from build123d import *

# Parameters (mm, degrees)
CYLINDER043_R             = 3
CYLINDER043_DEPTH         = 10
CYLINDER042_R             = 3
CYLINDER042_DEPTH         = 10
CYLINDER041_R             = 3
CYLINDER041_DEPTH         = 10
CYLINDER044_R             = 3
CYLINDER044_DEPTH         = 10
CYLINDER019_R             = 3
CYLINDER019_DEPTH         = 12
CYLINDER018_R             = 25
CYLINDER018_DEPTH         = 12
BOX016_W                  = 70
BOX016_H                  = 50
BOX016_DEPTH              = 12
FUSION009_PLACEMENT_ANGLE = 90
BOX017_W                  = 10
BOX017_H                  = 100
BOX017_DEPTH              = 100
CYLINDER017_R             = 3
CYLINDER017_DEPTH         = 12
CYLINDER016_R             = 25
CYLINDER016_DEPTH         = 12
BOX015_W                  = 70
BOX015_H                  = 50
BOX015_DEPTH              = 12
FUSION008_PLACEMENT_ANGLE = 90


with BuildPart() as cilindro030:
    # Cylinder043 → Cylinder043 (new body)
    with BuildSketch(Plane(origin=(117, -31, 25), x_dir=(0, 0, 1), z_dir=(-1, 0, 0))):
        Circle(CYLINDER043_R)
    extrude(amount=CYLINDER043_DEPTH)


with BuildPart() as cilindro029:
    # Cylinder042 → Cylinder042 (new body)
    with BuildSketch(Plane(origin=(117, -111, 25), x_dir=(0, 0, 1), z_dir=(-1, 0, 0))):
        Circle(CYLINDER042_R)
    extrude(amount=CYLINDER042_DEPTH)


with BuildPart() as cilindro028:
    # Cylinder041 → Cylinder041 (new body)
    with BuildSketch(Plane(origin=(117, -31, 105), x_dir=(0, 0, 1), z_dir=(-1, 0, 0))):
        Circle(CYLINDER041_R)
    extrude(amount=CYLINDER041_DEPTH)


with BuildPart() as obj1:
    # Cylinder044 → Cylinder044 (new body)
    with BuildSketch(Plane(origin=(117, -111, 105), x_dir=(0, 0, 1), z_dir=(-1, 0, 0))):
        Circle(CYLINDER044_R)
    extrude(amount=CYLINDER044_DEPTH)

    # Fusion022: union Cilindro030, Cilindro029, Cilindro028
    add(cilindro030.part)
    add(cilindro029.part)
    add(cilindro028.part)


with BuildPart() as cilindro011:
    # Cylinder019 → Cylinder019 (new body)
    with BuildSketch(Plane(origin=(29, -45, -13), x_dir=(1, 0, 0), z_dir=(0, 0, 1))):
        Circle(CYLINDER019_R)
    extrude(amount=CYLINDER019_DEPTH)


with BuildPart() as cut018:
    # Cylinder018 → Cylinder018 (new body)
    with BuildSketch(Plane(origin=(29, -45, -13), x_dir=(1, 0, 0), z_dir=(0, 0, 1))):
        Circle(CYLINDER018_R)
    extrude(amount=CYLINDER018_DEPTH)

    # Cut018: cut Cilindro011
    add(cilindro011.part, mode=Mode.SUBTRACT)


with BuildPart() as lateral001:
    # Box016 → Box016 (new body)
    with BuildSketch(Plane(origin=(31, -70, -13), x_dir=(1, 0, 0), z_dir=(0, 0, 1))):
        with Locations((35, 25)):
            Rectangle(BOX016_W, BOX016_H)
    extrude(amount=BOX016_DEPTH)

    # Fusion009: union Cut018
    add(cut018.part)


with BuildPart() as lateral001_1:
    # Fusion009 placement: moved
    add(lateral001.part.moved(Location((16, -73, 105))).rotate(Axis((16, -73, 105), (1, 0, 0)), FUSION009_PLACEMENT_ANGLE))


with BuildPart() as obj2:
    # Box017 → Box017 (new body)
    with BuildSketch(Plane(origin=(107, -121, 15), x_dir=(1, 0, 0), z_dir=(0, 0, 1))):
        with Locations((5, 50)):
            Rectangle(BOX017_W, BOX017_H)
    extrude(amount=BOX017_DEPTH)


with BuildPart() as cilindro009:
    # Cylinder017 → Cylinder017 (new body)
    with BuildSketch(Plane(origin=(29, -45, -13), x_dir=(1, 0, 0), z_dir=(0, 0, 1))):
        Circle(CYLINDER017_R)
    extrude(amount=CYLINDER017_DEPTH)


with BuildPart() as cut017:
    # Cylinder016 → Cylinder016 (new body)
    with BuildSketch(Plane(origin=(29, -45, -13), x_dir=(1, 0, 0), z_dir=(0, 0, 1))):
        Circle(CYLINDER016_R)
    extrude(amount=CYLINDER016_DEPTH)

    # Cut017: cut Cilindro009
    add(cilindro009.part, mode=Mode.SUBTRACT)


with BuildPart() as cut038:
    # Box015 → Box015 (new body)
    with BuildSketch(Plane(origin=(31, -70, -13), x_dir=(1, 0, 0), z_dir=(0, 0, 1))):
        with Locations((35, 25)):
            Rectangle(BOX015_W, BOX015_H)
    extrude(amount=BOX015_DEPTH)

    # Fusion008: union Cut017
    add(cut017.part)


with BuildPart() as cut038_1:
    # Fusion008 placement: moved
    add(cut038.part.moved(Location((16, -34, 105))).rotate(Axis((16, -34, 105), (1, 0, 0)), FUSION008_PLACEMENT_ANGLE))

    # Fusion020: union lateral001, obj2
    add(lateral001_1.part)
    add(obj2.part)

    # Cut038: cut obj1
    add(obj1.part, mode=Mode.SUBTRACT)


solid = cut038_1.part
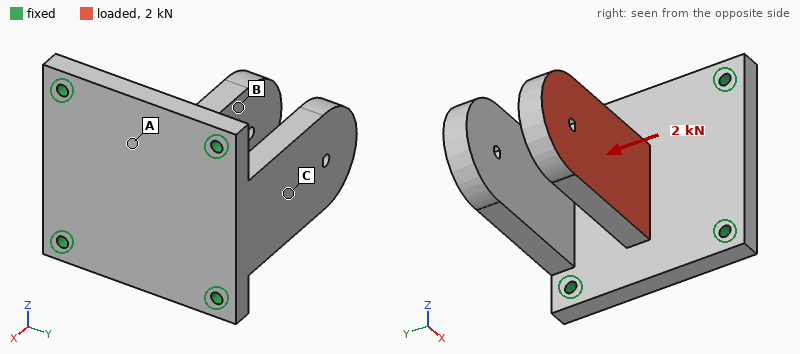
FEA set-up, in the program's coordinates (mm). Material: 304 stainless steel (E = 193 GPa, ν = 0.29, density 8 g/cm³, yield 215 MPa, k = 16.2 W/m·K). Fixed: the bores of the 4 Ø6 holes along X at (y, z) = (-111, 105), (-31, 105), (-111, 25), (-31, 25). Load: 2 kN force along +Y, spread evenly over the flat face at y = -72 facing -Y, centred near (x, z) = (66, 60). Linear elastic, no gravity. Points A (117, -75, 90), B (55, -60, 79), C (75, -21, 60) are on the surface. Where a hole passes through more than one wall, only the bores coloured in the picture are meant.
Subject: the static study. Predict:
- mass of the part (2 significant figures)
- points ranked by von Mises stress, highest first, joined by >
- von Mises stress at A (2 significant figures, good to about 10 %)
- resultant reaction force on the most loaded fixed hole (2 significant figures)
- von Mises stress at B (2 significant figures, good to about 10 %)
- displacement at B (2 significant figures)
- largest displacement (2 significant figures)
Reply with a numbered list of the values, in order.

1. 1.6 kg
2. A > B > C
3. 16 MPa
4. 1.0 kN
5. 9.5 MPa
6. 0.084 mm
7. 0.16 mm
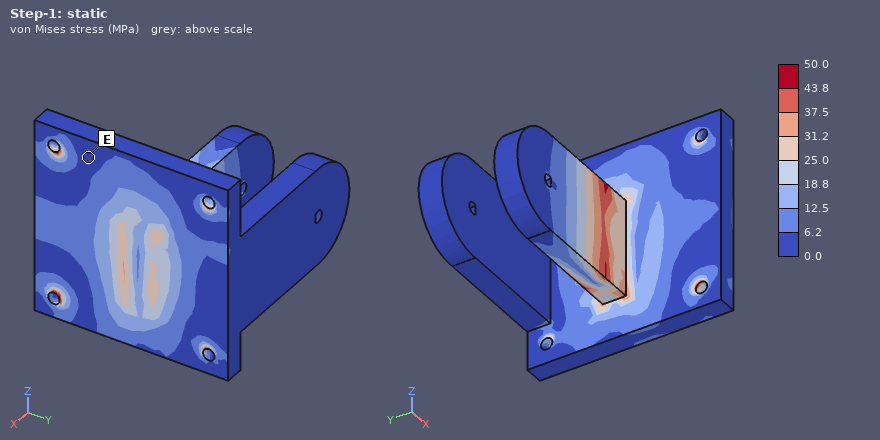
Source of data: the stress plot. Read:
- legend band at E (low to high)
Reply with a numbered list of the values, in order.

1. 0.0 to 6.2 MPa
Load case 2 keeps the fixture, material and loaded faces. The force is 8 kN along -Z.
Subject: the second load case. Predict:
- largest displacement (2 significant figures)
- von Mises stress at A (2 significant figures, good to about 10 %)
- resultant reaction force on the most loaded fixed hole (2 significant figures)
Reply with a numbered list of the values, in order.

1. 0.13 mm
2. 55 MPa
3. 4.0 kN
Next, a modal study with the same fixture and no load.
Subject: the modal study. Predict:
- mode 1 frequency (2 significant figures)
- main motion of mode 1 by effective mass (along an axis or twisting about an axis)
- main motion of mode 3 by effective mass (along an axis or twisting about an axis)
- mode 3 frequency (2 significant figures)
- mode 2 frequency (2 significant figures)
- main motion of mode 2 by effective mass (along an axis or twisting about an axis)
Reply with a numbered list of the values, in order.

1. 970 Hz
2. along Y
3. along Z
4. 2300 Hz
5. 1200 Hz
6. along Y
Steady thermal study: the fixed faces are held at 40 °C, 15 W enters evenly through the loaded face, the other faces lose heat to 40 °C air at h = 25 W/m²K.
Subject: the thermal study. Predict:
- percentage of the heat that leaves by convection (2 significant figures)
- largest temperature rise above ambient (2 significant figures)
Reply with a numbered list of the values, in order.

1. 65 %
2. 48 K
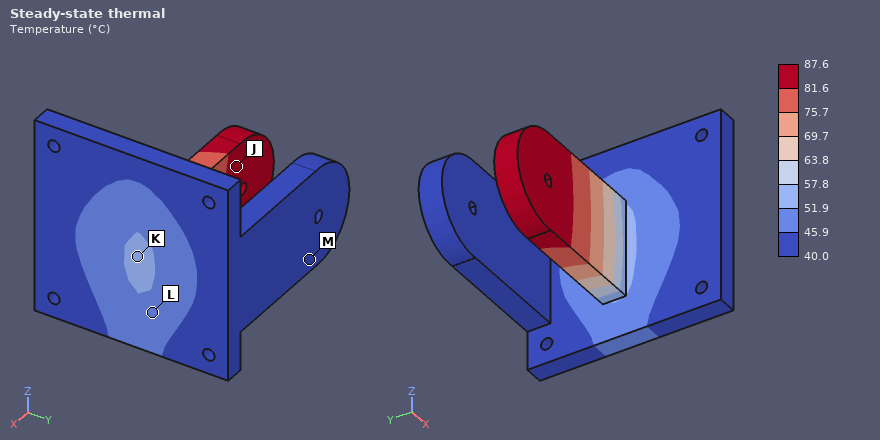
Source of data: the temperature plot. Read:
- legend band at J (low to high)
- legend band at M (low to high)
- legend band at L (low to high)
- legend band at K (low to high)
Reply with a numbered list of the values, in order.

1. 81.6 to 87.6 °C
2. 40.0 to 45.9 °C
3. 45.9 to 51.9 °C
4. 51.9 to 57.8 °C
